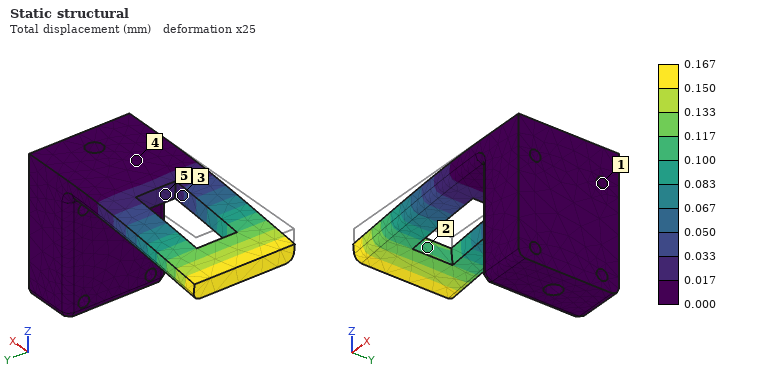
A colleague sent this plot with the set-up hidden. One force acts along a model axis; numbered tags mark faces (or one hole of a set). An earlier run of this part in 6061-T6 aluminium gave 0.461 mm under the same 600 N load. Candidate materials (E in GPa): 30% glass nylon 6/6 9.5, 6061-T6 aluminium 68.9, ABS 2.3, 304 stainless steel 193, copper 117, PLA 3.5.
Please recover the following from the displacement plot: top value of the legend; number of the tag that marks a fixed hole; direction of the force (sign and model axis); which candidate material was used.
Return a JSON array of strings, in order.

["0.167 mm", "1", "-Z", "304 stainless steel"]
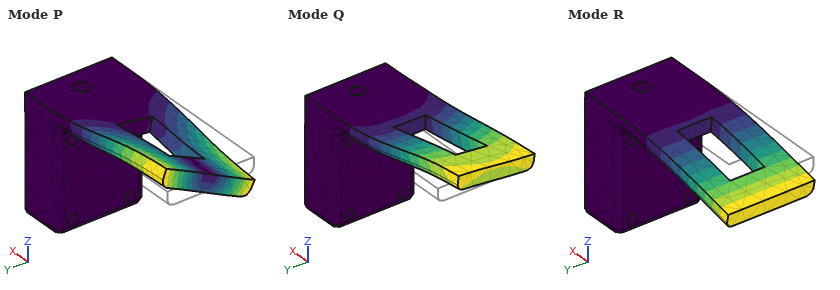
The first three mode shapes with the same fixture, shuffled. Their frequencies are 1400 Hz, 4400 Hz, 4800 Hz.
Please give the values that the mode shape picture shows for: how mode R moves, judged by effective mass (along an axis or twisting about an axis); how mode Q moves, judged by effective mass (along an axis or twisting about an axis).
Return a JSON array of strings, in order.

["along Z", "along Y"]
